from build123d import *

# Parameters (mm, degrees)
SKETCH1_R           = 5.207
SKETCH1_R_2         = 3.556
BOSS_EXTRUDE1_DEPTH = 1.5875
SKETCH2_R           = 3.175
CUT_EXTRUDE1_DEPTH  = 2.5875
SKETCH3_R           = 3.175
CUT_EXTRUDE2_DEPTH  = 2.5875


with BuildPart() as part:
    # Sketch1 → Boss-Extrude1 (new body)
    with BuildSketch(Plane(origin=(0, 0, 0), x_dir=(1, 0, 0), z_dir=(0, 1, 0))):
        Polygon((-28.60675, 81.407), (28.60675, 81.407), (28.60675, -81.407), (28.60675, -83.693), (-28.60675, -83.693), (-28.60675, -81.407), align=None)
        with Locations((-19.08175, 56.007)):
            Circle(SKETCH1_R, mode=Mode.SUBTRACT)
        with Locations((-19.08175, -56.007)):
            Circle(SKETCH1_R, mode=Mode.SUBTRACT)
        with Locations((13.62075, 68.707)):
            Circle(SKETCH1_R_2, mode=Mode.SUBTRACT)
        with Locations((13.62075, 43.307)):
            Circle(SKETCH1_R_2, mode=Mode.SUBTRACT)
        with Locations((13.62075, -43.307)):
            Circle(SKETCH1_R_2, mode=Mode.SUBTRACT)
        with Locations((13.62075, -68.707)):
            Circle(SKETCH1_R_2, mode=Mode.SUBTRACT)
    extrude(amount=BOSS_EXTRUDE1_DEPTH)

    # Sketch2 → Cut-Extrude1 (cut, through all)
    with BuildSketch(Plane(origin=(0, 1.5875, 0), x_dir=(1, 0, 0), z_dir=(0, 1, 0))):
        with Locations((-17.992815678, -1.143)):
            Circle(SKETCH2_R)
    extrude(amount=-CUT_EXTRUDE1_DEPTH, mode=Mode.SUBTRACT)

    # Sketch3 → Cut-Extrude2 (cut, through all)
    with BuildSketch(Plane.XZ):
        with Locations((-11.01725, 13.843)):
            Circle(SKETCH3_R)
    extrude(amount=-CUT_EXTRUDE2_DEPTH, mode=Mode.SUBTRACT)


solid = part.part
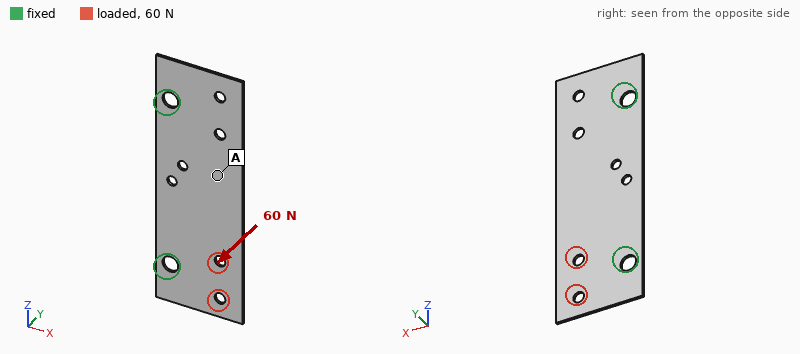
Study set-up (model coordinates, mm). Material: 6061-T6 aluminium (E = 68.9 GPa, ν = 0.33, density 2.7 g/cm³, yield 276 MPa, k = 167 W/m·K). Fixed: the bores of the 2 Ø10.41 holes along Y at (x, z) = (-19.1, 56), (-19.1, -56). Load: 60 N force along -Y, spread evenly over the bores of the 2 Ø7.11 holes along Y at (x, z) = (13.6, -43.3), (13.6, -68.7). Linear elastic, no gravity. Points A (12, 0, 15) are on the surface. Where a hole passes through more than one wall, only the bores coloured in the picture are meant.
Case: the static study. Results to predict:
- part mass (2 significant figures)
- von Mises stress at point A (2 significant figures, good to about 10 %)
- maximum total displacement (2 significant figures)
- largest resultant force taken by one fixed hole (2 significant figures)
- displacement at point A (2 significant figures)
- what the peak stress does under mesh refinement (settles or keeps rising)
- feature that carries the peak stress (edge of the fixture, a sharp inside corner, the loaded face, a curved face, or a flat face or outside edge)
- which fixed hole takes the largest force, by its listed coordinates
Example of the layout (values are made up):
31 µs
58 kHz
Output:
39 g
8.3 MPa
0.74 mm
59 N
0.17 mm
keeps rising
edge of the fixture
(-19.1, -56)
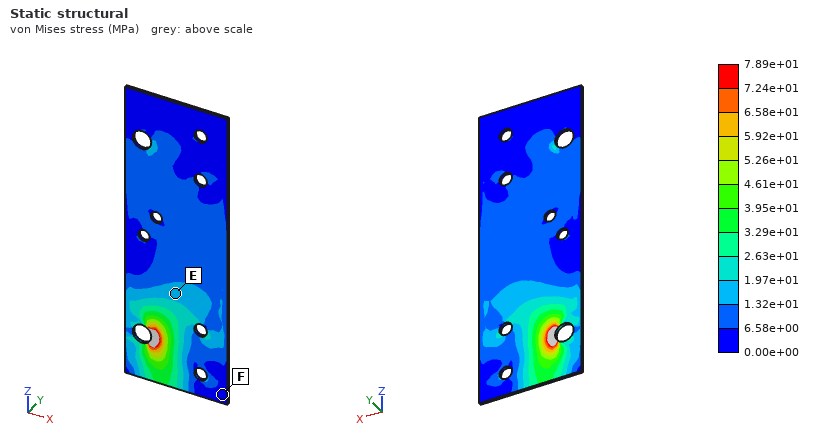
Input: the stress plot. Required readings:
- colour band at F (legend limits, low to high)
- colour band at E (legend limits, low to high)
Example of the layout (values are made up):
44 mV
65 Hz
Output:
0.00e+00 to 6.58e+00 MPa
1.32e+01 to 1.97e+01 MPa
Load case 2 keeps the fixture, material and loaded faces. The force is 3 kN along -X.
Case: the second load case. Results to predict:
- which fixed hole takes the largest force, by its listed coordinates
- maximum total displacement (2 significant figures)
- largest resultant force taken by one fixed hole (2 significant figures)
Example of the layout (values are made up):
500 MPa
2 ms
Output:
(-19.1, -56)
36 µm
3.0 kN
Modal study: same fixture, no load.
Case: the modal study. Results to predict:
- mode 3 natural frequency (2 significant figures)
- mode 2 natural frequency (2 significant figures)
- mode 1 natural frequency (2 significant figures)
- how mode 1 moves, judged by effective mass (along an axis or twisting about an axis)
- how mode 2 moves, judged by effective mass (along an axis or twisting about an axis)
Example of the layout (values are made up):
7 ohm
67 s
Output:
760 Hz
720 Hz
440 Hz
along Y
twisting about X
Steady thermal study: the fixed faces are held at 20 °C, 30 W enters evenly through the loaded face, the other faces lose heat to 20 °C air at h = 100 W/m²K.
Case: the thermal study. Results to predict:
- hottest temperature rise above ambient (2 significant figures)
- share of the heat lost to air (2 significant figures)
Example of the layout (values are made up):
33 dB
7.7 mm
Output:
48 K
59 %
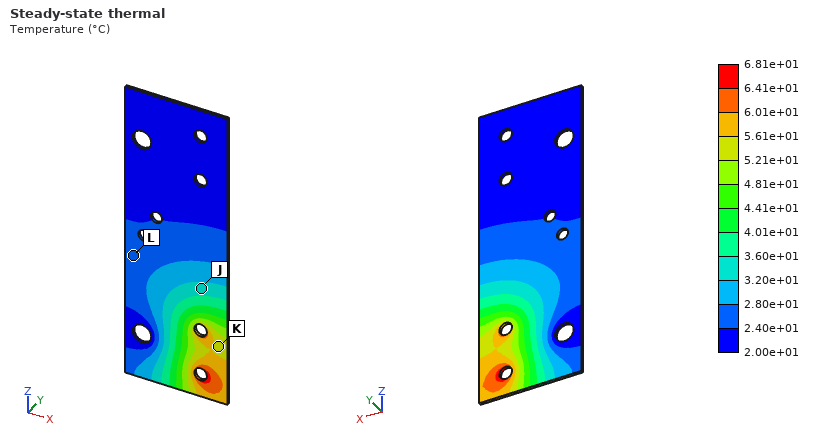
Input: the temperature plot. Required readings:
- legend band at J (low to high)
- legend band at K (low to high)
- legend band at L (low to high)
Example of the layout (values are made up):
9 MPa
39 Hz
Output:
3.20e+01 to 3.60e+01 °C
5.21e+01 to 5.61e+01 °C
2.40e+01 to 2.80e+01 °C
